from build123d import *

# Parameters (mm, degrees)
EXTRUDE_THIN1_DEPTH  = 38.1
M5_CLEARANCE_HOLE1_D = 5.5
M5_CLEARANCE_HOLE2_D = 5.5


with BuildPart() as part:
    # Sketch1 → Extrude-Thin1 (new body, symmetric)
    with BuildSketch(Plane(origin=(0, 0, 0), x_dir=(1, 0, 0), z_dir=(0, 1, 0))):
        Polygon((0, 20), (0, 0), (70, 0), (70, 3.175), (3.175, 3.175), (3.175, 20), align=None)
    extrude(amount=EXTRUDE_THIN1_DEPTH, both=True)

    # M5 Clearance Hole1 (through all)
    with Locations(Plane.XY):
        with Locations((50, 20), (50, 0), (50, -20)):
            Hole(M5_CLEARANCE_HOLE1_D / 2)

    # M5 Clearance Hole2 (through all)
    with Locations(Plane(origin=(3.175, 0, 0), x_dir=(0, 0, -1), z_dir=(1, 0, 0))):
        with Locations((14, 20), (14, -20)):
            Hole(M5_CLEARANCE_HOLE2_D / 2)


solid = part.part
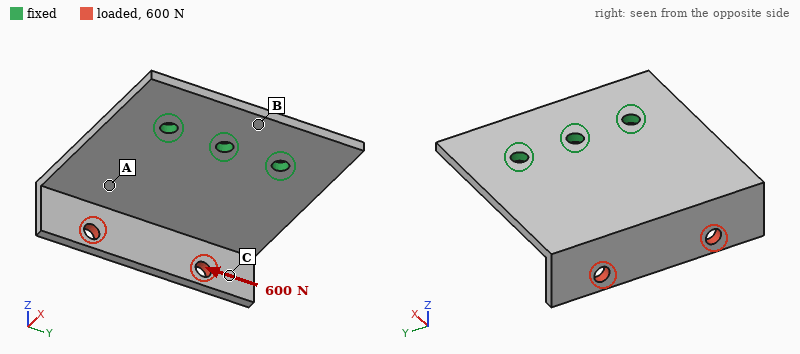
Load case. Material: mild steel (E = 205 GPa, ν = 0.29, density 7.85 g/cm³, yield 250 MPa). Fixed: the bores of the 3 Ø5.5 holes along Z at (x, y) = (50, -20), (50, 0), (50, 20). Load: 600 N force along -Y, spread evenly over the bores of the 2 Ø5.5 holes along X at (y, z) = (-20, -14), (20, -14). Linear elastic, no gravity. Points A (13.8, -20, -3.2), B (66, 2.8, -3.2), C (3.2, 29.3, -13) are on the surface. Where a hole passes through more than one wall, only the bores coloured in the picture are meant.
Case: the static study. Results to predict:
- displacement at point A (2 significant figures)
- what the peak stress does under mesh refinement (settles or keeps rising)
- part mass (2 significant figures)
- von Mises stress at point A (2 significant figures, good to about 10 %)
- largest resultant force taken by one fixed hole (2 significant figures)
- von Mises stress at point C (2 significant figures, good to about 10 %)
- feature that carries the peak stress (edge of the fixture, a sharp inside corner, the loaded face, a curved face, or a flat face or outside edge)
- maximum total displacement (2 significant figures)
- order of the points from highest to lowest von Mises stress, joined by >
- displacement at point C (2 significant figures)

0.046 mm
keeps rising
160 g
38 MPa
710 N
17 MPa
edge of the fixture
0.14 mm
A > C > B
0.100 mm
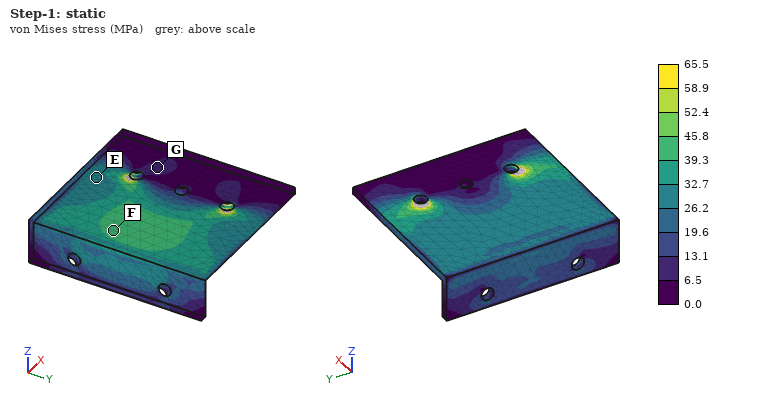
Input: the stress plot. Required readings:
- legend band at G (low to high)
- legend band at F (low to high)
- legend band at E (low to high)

6.5 to 13.1 MPa
39.3 to 45.8 MPa
26.2 to 32.7 MPa
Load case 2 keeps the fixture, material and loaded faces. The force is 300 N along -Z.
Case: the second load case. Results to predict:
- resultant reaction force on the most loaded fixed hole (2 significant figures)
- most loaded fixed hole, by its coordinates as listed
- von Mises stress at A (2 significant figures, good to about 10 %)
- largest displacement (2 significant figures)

120 N
(50, 0)
26 MPa
0.30 mm
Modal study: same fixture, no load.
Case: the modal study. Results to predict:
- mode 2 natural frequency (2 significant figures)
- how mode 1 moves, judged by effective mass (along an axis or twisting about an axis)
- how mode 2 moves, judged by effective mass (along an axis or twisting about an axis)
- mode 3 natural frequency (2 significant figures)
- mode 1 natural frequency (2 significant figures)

1300 Hz
along Z
twisting about X
3600 Hz
710 Hz
